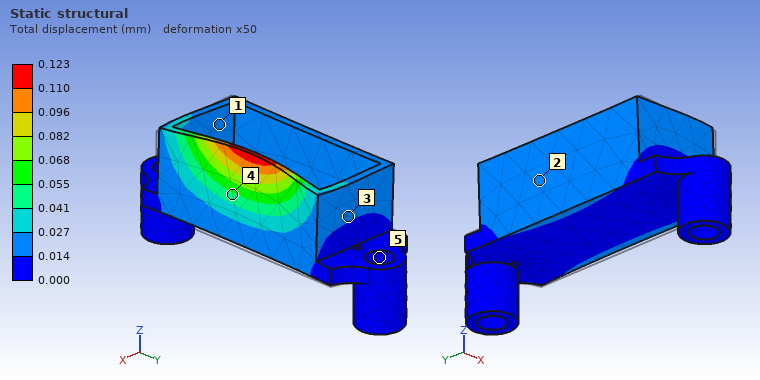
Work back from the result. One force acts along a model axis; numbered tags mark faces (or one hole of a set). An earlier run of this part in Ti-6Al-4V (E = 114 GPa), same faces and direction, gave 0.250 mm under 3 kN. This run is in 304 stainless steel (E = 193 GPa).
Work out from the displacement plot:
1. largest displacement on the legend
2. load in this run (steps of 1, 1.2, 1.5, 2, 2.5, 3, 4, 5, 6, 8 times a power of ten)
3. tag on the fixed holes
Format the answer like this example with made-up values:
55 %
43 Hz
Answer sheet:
0.123 mm
2.5 kN
5
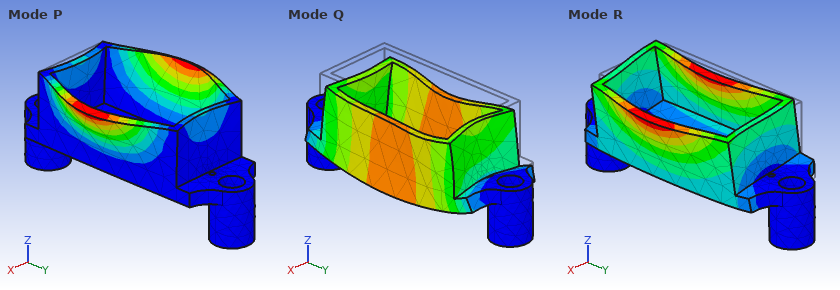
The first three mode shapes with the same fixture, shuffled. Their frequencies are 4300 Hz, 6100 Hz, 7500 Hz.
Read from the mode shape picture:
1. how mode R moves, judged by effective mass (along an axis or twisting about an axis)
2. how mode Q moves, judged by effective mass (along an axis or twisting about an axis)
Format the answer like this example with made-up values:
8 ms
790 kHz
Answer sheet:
along X
along Z
